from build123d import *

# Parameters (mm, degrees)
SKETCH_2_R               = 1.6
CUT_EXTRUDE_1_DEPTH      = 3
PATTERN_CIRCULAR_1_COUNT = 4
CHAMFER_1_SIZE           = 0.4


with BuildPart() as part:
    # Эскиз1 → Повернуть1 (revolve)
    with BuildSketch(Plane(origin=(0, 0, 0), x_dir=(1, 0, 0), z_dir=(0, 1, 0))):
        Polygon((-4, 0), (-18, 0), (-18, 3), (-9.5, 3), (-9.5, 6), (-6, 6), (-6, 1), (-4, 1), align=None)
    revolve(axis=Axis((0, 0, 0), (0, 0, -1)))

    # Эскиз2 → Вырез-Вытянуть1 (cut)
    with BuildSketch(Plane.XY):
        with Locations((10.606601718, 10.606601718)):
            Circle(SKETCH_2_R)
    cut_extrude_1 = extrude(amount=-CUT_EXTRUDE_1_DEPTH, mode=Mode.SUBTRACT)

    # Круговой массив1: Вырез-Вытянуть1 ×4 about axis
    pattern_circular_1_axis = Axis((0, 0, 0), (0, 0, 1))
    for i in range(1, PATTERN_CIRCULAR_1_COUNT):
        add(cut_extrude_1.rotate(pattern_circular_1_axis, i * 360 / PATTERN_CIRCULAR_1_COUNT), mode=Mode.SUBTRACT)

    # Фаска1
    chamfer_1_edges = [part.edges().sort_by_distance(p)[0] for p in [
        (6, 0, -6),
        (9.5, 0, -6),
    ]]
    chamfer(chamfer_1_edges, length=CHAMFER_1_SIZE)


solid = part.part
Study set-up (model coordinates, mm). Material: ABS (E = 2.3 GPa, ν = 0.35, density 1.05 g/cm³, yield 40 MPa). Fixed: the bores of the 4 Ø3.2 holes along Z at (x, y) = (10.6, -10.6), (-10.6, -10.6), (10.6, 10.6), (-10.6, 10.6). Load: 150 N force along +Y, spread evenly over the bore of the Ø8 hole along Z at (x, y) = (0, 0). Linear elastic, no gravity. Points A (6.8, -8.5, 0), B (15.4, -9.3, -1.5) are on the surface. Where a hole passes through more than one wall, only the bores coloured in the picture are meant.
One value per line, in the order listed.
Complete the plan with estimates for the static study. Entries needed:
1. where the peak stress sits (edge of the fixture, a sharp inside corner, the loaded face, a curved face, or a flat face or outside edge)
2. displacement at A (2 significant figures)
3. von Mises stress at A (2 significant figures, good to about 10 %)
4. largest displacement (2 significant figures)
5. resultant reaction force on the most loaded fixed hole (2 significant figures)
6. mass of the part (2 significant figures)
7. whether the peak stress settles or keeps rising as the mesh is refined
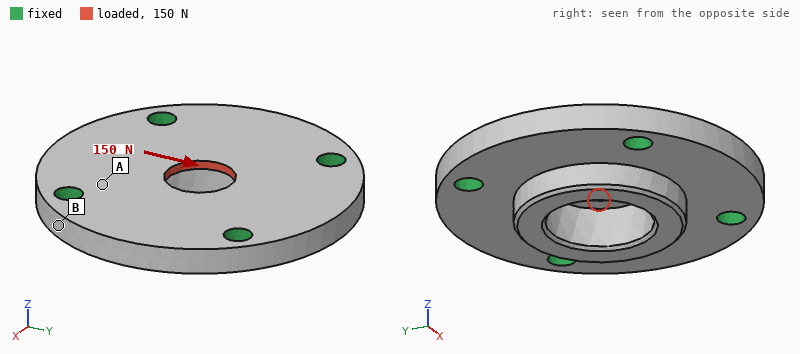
a sharp inside corner
4.2 µm
2.2 MPa
22 µm
39 N
3.3 g
keeps rising
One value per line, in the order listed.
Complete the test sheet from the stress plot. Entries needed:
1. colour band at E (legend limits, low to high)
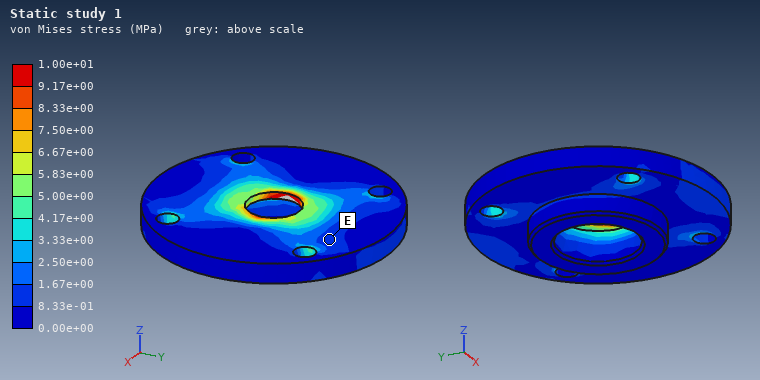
8.33e-01 to 1.67e+00 MPa
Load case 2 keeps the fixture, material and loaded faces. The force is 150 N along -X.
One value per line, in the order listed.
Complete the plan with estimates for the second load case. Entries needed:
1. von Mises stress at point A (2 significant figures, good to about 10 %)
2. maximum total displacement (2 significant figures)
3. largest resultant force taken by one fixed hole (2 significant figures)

2.0 MPa
22 µm
39 N
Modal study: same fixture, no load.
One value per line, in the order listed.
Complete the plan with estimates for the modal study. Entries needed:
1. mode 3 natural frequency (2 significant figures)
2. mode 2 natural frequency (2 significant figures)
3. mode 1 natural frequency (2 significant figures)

8900 Hz
8600 Hz
8600 Hz
